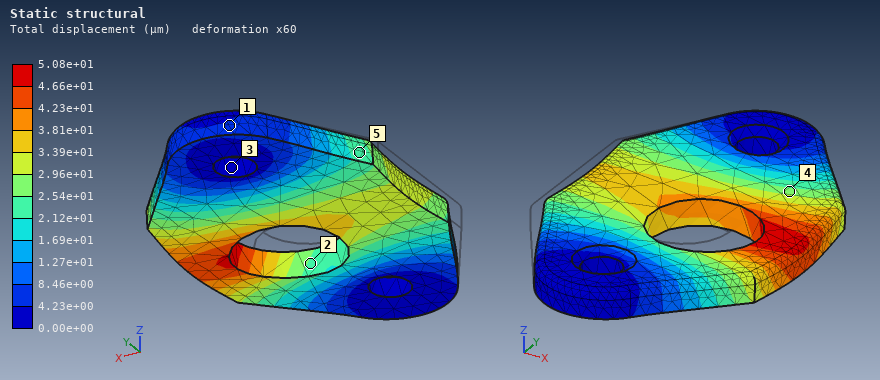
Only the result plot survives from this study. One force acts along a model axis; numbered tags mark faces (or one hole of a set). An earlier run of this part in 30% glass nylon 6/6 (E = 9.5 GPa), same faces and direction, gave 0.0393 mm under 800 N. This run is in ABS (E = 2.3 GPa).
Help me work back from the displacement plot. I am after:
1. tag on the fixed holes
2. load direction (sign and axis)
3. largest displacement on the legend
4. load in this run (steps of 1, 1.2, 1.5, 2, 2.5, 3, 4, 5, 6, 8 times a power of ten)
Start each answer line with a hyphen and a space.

- 3
- +X
- 5.08e+01 µm
- 250 N
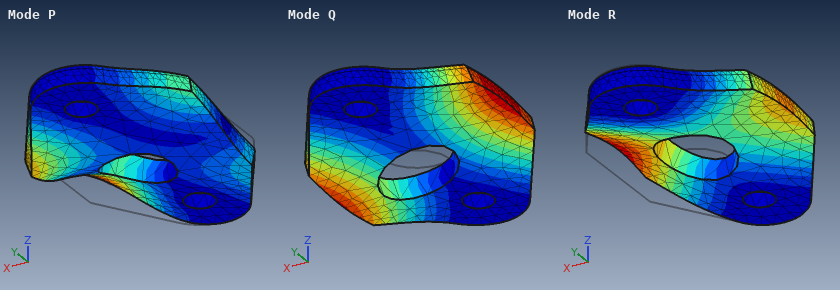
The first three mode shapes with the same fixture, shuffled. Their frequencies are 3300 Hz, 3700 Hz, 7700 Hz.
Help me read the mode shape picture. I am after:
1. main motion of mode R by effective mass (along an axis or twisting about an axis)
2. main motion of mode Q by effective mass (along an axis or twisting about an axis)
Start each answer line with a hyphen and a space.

- along Z
- twisting about Y
